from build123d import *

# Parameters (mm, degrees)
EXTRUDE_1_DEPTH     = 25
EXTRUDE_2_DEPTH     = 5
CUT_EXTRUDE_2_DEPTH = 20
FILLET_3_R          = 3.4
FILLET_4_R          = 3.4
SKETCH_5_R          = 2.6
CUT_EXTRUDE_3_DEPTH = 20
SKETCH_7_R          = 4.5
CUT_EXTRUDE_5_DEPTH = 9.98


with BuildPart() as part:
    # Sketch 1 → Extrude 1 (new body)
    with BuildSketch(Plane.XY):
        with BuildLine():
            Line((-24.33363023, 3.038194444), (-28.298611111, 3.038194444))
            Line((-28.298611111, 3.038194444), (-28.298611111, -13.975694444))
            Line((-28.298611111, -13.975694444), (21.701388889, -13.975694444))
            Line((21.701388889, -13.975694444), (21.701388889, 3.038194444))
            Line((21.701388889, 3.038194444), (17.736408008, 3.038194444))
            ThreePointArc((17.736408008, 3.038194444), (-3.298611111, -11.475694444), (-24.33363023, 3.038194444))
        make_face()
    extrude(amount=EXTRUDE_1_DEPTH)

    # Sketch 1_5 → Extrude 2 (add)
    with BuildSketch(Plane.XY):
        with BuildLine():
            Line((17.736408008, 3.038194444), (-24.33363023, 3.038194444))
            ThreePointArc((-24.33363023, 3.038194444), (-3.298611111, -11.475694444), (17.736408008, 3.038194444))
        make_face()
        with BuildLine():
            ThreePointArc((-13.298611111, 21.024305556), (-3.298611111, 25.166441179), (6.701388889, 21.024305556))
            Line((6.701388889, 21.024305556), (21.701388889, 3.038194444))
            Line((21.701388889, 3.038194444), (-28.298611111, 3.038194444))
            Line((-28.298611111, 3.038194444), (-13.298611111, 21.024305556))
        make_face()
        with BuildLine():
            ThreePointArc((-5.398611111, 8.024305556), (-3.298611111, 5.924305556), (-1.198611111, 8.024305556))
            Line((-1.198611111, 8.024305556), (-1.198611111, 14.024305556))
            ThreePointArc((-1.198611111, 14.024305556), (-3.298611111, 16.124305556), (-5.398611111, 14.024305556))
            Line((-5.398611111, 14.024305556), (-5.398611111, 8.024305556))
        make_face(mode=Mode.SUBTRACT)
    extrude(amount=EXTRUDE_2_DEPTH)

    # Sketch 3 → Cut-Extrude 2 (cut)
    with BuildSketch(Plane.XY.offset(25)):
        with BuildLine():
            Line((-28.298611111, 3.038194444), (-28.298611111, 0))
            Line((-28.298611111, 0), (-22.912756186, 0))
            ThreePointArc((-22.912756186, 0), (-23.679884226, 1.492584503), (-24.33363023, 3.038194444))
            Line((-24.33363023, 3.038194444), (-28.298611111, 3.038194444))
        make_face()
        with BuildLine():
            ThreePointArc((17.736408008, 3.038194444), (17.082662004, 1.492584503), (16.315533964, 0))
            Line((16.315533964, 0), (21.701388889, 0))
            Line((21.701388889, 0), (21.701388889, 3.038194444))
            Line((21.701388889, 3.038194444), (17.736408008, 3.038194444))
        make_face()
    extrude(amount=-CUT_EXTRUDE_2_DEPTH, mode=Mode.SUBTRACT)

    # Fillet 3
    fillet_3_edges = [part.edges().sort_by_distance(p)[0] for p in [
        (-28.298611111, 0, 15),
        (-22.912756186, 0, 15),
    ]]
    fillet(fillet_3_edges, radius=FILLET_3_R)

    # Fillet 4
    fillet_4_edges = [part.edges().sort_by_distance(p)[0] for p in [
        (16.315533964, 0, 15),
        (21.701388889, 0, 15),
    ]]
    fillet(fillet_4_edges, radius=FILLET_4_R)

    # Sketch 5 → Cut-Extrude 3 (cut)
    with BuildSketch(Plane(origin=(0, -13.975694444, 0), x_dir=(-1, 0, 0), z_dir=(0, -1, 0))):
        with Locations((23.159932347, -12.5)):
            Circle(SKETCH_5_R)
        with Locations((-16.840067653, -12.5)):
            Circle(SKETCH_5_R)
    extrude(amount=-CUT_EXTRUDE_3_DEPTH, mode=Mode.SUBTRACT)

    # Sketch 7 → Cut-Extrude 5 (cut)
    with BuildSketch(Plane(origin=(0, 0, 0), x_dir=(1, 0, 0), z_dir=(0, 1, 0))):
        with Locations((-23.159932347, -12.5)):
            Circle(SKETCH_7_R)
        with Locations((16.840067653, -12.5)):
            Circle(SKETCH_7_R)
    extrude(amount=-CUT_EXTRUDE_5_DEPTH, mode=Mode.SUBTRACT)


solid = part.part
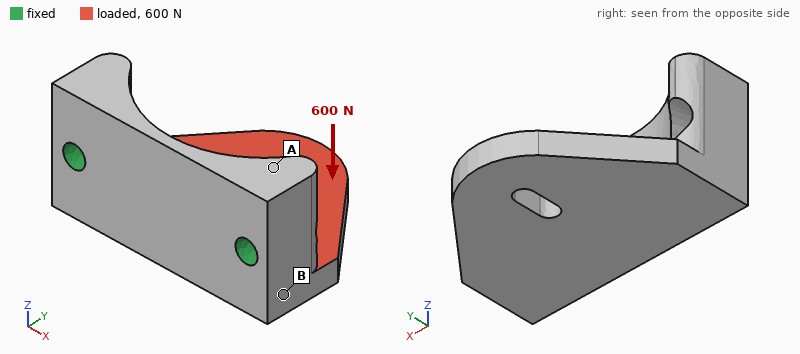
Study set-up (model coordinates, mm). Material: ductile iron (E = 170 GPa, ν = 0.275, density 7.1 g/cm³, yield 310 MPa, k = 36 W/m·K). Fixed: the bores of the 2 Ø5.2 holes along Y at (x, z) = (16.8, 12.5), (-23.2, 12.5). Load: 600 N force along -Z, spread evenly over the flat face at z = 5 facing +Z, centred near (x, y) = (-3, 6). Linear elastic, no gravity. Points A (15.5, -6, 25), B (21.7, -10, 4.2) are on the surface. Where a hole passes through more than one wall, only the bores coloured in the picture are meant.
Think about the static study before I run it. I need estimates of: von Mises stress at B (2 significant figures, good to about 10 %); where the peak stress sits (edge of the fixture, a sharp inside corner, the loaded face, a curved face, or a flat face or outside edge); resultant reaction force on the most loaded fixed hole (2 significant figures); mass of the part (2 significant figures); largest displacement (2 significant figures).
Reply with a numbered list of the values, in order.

1. 19 MPa
2. a curved face
3. 300 N
4. 97 g
5. 57 µm
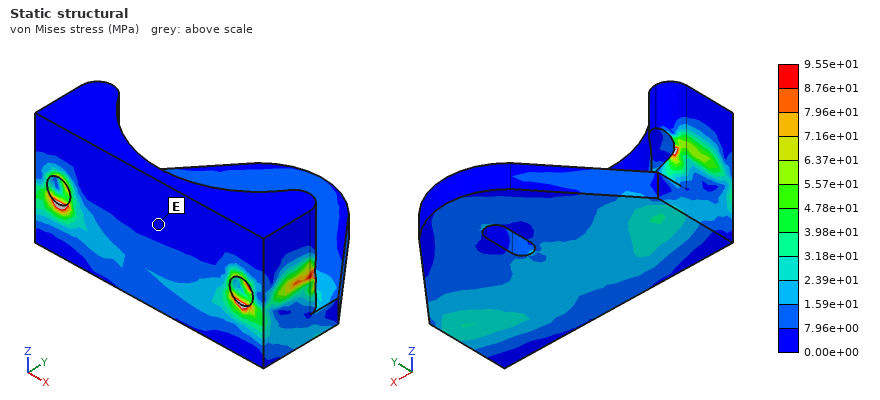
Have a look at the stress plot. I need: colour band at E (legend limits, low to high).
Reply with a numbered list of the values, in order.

1. 0.00e+00 to 7.96e+00 MPa
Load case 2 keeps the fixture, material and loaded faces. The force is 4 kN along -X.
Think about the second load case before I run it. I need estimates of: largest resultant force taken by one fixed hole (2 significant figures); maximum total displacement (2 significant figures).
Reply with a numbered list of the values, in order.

1. 2.6 kN
2. 35 µm
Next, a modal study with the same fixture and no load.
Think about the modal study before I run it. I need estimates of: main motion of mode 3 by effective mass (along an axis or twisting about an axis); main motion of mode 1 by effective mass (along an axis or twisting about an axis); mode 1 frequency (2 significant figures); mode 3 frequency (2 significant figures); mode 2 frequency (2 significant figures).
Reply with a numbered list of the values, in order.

1. along Y
2. along Z
3. 3400 Hz
4. 10 kHz
5. 8500 Hz
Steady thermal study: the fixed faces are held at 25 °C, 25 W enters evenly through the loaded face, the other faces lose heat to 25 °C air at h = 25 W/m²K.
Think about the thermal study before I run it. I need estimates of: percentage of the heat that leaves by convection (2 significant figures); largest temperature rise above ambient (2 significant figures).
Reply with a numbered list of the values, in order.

1. 15 %
2. 73 K
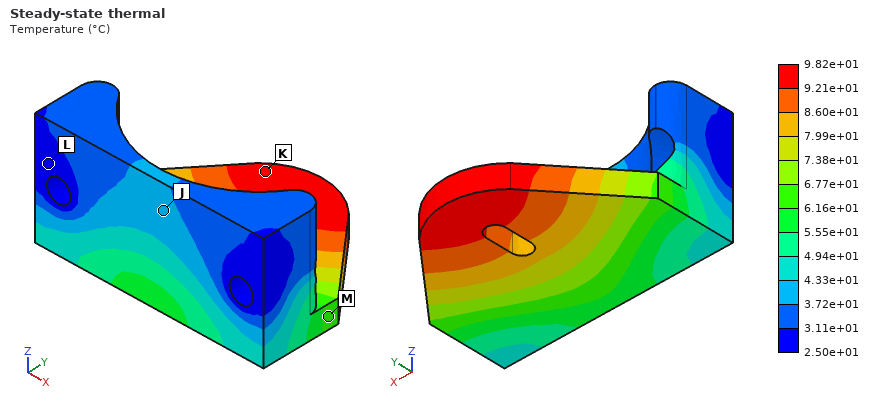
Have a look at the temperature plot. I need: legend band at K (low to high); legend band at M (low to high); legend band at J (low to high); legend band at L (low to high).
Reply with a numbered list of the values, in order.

1. 9.21e+01 to 9.82e+01 °C
2. 6.16e+01 to 6.77e+01 °C
3. 3.72e+01 to 4.33e+01 °C
4. 2.50e+01 to 3.11e+01 °C
